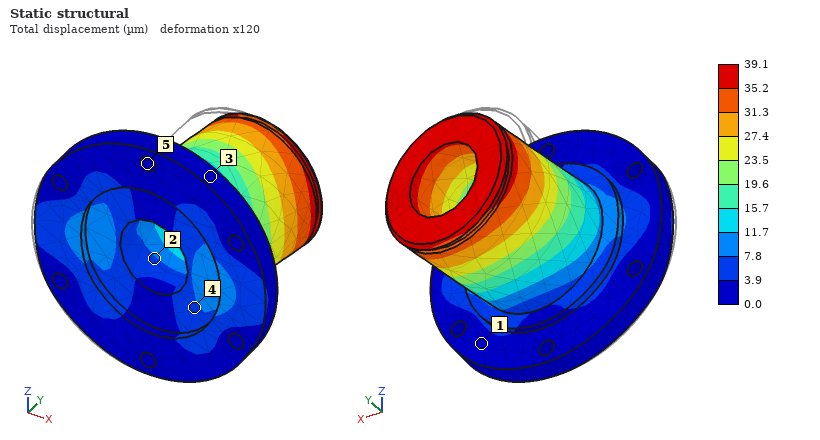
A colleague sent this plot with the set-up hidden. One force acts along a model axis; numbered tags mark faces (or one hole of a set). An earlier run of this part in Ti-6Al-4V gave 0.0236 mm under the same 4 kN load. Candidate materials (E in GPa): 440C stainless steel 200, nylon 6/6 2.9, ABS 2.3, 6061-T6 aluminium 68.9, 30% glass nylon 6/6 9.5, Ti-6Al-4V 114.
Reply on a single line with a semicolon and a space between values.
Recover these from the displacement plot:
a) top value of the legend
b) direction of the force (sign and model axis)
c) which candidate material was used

39.1 µm; +X; 6061-T6 aluminium
